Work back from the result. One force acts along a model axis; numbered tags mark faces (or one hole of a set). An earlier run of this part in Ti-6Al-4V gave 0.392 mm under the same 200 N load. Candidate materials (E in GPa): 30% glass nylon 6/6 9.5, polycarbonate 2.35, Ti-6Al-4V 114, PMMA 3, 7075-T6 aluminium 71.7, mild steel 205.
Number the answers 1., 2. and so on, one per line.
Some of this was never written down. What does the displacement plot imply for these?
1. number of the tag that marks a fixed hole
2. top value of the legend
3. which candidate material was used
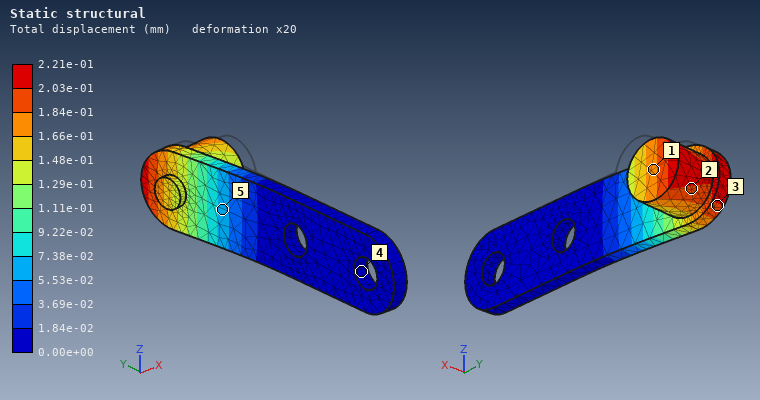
1. 4
2. 2.21e-01 mm
3. mild steel
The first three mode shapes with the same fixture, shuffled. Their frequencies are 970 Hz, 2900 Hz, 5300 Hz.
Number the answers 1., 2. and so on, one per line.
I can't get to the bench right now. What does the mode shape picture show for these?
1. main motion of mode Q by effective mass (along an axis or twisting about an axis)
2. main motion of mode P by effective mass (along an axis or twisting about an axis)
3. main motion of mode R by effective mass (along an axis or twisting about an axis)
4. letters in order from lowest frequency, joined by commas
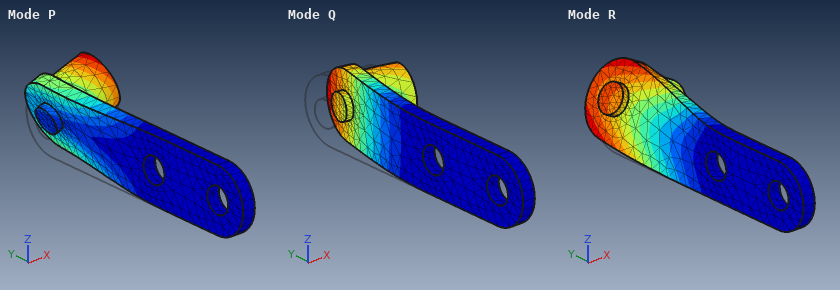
1. along X
2. along Z
3. along Z
4. Q, P, R
